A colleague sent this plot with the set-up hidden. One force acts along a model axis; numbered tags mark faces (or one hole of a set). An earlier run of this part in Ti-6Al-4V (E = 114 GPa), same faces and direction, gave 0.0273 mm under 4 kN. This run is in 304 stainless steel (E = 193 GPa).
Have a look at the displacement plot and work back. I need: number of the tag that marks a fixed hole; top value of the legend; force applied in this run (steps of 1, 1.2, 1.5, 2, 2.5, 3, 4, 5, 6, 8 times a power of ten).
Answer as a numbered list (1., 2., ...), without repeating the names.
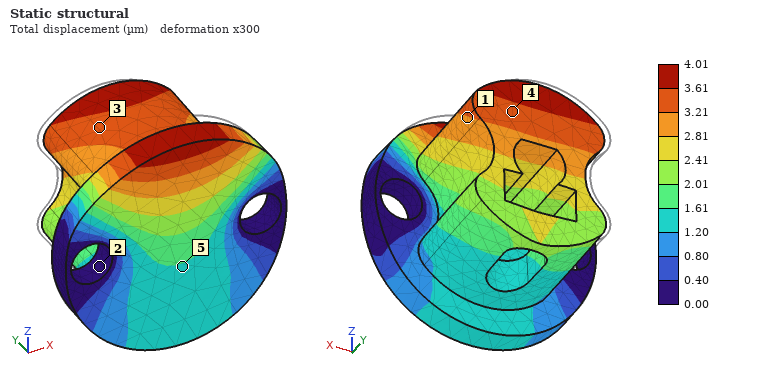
1. 2
2. 4.01 µm
3. 1 kN
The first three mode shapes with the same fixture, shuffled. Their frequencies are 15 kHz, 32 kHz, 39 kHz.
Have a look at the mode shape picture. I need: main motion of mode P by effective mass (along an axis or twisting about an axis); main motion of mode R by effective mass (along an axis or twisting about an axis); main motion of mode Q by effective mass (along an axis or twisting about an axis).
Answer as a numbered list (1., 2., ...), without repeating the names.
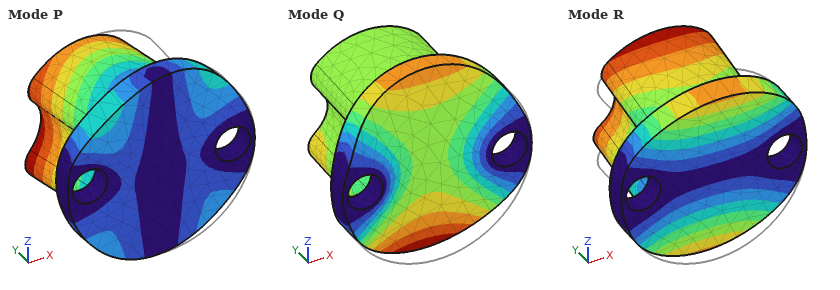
1. along X
2. along Z
3. along Y
